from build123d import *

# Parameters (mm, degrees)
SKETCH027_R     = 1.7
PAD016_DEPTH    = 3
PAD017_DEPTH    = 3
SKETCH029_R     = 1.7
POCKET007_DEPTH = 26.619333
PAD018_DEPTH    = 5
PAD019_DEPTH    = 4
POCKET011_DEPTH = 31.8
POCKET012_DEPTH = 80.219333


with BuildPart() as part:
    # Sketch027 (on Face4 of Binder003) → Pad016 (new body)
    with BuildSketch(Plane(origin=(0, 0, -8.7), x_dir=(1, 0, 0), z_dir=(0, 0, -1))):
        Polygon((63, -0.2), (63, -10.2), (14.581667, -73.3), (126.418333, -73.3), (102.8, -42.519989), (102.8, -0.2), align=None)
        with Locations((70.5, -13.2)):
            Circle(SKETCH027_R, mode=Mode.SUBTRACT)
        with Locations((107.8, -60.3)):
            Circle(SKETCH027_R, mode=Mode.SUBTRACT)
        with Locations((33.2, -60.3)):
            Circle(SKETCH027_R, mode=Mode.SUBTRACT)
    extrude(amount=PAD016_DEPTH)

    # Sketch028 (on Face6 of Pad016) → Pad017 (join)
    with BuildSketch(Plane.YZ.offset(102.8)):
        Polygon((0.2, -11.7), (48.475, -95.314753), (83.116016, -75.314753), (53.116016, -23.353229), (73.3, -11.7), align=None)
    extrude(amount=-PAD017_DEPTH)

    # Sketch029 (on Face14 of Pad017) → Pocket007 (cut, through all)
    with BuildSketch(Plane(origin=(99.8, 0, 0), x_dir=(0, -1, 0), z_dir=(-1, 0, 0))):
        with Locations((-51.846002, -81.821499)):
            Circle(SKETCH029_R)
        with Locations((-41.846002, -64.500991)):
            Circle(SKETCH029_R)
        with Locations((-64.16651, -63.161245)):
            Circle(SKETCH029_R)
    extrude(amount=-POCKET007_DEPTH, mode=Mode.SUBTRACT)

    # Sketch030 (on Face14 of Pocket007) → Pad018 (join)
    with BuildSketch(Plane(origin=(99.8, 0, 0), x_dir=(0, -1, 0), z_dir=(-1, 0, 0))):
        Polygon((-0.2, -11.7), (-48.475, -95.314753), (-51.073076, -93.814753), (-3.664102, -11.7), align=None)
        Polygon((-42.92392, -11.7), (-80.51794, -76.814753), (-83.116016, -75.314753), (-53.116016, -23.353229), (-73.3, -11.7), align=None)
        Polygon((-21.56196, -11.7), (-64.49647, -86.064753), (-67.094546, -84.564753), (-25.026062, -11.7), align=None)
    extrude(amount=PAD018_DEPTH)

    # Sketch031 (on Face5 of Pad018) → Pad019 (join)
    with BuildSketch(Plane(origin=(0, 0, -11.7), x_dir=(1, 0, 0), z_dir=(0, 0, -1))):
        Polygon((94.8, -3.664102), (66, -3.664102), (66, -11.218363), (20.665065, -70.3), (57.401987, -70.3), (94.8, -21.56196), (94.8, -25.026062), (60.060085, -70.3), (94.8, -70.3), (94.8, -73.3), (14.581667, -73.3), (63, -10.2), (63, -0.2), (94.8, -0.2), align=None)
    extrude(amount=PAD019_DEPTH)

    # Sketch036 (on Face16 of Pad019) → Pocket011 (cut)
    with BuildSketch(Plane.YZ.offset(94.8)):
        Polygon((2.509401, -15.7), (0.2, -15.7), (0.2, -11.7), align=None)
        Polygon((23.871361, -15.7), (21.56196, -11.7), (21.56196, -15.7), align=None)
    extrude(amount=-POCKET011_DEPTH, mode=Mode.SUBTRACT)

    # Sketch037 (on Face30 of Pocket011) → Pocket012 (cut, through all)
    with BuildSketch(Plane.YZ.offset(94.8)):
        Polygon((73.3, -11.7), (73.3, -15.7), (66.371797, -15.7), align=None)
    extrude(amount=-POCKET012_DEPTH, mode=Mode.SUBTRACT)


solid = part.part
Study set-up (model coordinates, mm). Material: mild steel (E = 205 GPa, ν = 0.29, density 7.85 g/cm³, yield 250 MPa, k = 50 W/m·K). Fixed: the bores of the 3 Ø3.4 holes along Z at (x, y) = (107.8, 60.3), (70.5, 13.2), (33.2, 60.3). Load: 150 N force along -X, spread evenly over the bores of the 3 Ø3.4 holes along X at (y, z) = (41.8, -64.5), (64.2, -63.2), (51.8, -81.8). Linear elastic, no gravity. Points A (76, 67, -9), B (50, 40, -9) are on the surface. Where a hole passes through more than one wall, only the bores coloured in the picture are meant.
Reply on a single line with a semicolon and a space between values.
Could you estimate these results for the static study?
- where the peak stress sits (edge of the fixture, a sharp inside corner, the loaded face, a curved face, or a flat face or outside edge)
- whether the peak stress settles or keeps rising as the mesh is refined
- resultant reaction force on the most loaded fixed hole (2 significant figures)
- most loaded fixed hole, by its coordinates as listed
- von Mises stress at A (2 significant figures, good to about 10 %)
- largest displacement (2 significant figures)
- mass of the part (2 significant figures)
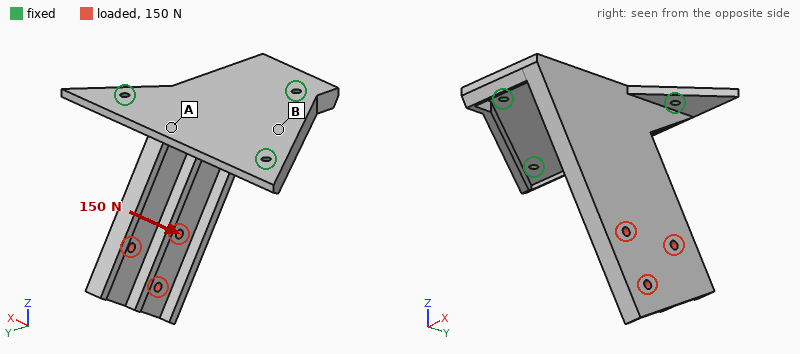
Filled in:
edge of the fixture; keeps rising; 190 N; (107.8, 60.3); 17 MPa; 0.31 mm; 250 g
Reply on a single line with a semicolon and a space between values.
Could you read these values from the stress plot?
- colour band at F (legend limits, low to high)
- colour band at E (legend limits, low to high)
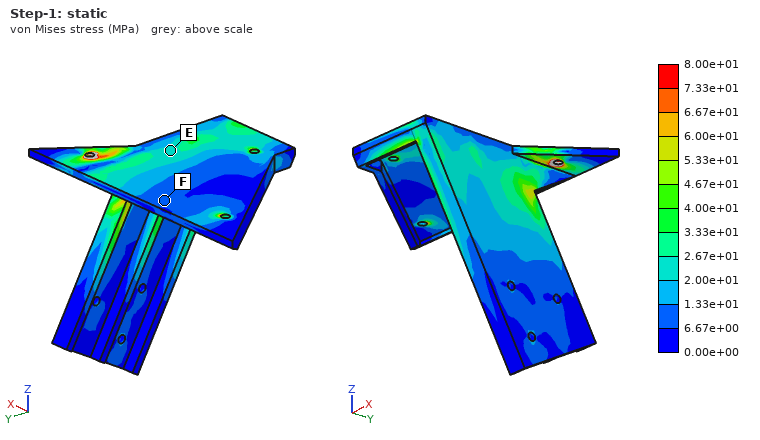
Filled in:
6.67e+00 to 1.33e+01 MPa; 2.00e+01 to 2.67e+01 MPa
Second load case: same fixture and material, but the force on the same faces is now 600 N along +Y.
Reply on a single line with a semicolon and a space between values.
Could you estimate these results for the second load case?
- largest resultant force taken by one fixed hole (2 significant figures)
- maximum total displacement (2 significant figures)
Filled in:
590 N; 0.39 mm
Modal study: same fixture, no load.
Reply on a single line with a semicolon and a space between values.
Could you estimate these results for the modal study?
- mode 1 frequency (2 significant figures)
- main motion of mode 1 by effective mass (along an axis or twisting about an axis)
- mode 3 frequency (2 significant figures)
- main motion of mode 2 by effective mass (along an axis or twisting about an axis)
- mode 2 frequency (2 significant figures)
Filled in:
570 Hz; along X; 1900 Hz; along Y; 1200 Hz
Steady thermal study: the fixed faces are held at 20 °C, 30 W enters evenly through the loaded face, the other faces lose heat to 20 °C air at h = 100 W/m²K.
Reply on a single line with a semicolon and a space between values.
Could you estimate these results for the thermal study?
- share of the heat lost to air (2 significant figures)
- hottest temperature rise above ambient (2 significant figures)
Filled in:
95 %; 69 K
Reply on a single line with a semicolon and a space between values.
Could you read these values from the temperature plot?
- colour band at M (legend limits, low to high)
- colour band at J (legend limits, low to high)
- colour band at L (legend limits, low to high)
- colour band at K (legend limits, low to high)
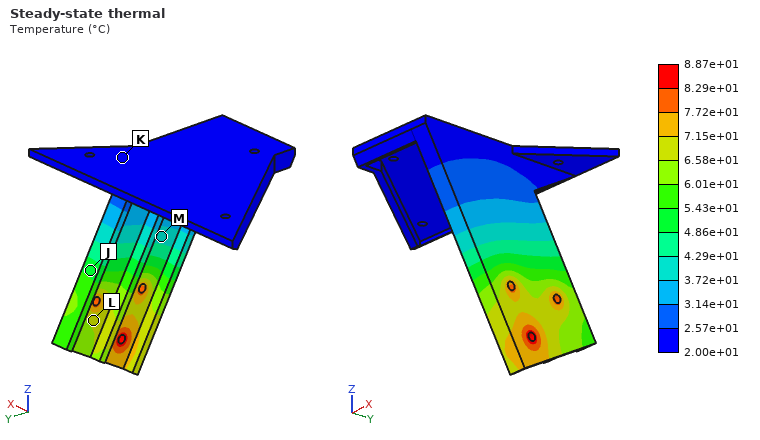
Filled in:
3.72e+01 to 4.29e+01 °C; 4.86e+01 to 5.43e+01 °C; 6.58e+01 to 7.15e+01 °C; 2.00e+01 to 2.57e+01 °C
